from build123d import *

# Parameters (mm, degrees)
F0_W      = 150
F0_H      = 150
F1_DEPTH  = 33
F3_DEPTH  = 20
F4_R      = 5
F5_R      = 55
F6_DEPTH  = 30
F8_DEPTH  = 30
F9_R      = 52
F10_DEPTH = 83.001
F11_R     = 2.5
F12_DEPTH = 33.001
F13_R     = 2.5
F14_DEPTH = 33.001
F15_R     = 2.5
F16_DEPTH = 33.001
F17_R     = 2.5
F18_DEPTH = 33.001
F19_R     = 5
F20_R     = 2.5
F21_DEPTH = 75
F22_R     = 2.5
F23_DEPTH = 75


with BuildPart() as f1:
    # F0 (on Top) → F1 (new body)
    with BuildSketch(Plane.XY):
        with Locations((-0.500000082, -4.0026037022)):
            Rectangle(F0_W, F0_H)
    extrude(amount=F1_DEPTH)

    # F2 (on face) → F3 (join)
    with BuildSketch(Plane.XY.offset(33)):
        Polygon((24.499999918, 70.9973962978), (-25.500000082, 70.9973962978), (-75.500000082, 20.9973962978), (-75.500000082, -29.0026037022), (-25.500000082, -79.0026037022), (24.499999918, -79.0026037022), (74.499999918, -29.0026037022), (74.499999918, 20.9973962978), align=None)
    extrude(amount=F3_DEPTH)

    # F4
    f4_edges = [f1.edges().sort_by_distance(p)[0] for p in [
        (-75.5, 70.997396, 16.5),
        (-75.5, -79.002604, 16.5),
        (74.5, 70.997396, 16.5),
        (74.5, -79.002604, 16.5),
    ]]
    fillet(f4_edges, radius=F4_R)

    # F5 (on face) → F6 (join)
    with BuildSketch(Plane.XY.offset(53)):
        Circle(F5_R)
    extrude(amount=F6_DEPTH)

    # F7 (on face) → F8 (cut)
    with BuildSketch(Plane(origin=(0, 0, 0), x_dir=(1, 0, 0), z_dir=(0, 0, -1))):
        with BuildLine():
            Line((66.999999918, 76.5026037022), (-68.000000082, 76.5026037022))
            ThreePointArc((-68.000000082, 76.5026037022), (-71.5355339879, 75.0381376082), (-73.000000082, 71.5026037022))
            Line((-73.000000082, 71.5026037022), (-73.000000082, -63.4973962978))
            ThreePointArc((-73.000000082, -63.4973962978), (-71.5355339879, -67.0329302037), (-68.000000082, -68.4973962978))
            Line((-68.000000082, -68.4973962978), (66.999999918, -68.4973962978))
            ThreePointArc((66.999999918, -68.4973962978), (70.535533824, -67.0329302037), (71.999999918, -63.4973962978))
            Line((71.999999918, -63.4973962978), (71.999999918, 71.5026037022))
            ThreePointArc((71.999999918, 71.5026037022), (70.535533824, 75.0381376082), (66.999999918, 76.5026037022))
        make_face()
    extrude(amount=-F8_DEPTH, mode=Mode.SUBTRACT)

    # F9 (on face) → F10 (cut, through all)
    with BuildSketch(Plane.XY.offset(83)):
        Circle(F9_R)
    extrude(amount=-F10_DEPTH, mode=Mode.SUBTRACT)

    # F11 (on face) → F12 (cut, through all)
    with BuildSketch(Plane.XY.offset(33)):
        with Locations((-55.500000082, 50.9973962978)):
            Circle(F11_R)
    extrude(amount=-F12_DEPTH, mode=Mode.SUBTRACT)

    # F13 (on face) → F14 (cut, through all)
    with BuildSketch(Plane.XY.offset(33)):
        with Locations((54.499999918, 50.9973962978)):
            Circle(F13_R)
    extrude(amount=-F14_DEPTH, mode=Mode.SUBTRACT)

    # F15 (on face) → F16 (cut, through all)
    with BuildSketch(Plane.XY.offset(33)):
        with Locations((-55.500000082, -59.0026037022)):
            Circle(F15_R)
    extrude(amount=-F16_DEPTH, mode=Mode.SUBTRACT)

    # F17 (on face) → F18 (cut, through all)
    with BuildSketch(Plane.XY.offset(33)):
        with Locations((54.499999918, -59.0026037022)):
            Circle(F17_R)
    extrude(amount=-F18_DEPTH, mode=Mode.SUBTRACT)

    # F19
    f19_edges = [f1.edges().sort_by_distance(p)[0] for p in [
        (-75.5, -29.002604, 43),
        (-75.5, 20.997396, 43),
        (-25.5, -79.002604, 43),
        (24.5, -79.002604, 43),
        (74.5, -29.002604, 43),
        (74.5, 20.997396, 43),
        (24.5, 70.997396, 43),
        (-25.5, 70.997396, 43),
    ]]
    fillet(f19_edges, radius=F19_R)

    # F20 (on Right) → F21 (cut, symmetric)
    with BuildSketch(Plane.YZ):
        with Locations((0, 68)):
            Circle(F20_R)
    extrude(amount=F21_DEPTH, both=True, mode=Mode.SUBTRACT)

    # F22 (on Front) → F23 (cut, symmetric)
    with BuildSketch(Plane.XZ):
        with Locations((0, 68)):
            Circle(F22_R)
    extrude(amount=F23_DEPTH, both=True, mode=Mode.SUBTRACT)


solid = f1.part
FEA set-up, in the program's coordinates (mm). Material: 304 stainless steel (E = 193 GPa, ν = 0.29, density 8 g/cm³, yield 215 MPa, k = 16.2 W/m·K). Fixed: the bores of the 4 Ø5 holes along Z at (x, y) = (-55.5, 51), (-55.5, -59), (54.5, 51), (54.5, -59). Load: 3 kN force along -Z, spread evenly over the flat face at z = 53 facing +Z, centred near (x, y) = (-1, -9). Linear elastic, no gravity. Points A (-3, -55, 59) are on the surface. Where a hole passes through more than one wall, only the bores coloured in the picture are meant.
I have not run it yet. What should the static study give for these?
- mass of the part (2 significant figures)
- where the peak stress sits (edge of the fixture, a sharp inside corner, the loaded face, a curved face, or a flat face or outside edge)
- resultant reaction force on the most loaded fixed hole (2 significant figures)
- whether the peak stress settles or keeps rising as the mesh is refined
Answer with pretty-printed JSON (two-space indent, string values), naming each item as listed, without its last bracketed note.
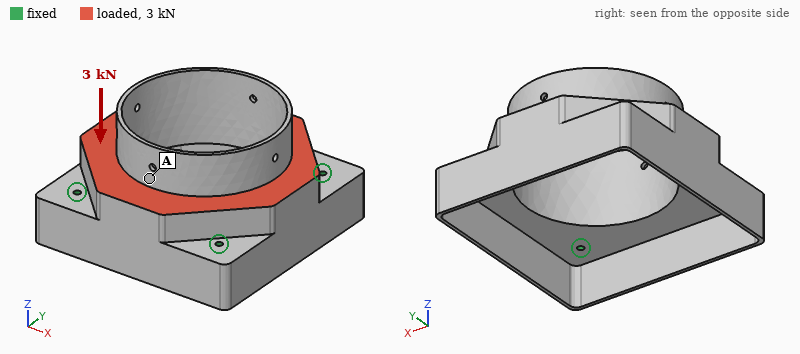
{
  "mass of the part": "2.4 kg",
  "where the peak stress sits": "edge of the fixture",
  "resultant reaction force on the most loaded fixed hole": "900 N",
  "whether the peak stress settles or keeps rising as the mesh is refined": "keeps rising"
}
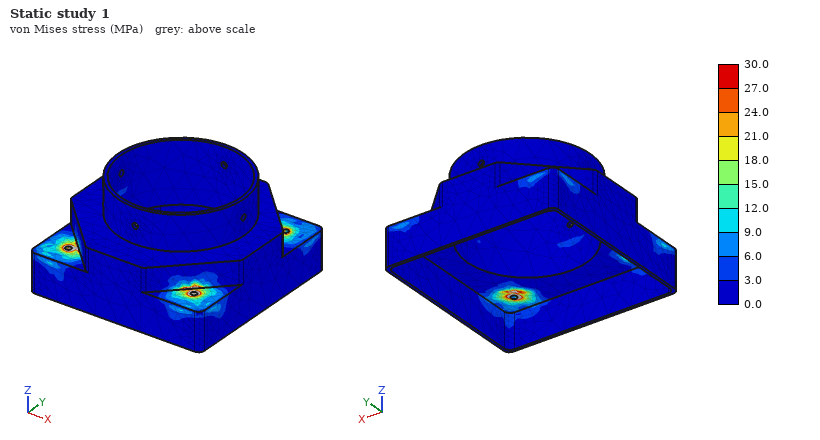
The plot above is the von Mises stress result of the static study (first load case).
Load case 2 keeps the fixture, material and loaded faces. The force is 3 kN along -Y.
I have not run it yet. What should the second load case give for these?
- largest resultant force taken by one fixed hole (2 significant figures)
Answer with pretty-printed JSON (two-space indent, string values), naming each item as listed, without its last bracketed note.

{
  "largest resultant force taken by one fixed hole": "850 N"
}
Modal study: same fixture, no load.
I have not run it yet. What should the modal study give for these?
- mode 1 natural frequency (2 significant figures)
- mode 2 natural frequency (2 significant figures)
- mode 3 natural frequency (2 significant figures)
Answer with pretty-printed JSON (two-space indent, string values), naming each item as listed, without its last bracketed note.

{
  "mode 1 natural frequency": "2200 Hz",
  "mode 2 natural frequency": "2300 Hz",
  "mode 3 natural frequency": "2300 Hz"
}
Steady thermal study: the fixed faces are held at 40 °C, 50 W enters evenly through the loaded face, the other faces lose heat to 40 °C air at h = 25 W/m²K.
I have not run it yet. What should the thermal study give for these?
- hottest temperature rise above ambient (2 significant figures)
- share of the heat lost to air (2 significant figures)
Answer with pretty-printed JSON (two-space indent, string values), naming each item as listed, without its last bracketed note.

{
  "hottest temperature rise above ambient": "33 K",
  "share of the heat lost to air": "79 %"
}
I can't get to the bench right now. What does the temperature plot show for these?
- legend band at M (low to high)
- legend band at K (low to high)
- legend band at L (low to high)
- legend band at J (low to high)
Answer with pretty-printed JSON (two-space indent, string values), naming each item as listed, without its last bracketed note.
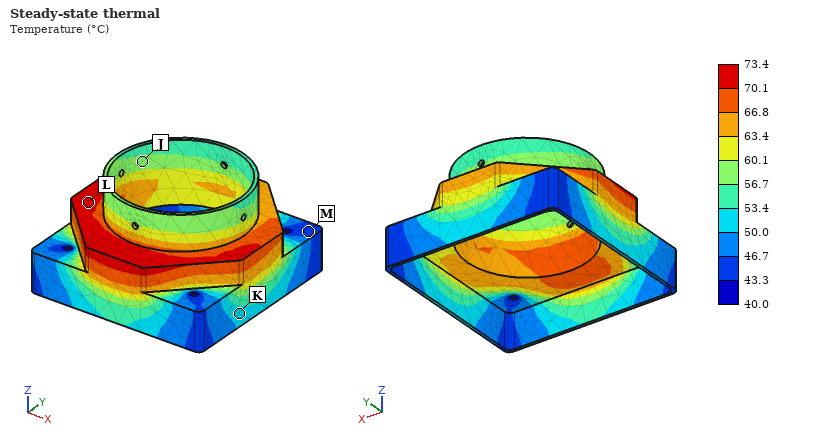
{
  "legend band at M": "43.3 to 46.7 °C",
  "legend band at K": "50.0 to 53.4 °C",
  "legend band at L": "70.1 to 73.4 °C",
  "legend band at J": "56.7 to 60.1 °C"
}
